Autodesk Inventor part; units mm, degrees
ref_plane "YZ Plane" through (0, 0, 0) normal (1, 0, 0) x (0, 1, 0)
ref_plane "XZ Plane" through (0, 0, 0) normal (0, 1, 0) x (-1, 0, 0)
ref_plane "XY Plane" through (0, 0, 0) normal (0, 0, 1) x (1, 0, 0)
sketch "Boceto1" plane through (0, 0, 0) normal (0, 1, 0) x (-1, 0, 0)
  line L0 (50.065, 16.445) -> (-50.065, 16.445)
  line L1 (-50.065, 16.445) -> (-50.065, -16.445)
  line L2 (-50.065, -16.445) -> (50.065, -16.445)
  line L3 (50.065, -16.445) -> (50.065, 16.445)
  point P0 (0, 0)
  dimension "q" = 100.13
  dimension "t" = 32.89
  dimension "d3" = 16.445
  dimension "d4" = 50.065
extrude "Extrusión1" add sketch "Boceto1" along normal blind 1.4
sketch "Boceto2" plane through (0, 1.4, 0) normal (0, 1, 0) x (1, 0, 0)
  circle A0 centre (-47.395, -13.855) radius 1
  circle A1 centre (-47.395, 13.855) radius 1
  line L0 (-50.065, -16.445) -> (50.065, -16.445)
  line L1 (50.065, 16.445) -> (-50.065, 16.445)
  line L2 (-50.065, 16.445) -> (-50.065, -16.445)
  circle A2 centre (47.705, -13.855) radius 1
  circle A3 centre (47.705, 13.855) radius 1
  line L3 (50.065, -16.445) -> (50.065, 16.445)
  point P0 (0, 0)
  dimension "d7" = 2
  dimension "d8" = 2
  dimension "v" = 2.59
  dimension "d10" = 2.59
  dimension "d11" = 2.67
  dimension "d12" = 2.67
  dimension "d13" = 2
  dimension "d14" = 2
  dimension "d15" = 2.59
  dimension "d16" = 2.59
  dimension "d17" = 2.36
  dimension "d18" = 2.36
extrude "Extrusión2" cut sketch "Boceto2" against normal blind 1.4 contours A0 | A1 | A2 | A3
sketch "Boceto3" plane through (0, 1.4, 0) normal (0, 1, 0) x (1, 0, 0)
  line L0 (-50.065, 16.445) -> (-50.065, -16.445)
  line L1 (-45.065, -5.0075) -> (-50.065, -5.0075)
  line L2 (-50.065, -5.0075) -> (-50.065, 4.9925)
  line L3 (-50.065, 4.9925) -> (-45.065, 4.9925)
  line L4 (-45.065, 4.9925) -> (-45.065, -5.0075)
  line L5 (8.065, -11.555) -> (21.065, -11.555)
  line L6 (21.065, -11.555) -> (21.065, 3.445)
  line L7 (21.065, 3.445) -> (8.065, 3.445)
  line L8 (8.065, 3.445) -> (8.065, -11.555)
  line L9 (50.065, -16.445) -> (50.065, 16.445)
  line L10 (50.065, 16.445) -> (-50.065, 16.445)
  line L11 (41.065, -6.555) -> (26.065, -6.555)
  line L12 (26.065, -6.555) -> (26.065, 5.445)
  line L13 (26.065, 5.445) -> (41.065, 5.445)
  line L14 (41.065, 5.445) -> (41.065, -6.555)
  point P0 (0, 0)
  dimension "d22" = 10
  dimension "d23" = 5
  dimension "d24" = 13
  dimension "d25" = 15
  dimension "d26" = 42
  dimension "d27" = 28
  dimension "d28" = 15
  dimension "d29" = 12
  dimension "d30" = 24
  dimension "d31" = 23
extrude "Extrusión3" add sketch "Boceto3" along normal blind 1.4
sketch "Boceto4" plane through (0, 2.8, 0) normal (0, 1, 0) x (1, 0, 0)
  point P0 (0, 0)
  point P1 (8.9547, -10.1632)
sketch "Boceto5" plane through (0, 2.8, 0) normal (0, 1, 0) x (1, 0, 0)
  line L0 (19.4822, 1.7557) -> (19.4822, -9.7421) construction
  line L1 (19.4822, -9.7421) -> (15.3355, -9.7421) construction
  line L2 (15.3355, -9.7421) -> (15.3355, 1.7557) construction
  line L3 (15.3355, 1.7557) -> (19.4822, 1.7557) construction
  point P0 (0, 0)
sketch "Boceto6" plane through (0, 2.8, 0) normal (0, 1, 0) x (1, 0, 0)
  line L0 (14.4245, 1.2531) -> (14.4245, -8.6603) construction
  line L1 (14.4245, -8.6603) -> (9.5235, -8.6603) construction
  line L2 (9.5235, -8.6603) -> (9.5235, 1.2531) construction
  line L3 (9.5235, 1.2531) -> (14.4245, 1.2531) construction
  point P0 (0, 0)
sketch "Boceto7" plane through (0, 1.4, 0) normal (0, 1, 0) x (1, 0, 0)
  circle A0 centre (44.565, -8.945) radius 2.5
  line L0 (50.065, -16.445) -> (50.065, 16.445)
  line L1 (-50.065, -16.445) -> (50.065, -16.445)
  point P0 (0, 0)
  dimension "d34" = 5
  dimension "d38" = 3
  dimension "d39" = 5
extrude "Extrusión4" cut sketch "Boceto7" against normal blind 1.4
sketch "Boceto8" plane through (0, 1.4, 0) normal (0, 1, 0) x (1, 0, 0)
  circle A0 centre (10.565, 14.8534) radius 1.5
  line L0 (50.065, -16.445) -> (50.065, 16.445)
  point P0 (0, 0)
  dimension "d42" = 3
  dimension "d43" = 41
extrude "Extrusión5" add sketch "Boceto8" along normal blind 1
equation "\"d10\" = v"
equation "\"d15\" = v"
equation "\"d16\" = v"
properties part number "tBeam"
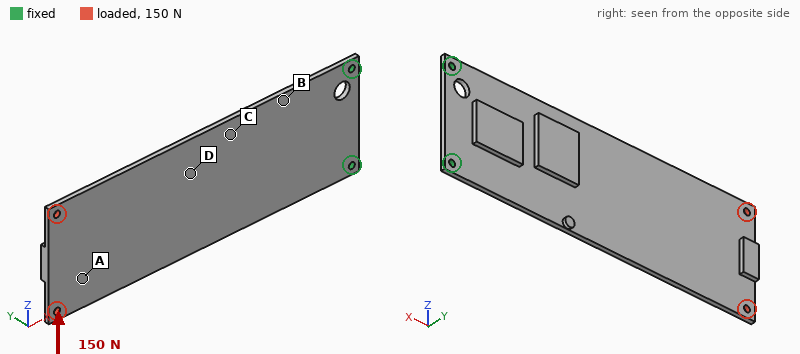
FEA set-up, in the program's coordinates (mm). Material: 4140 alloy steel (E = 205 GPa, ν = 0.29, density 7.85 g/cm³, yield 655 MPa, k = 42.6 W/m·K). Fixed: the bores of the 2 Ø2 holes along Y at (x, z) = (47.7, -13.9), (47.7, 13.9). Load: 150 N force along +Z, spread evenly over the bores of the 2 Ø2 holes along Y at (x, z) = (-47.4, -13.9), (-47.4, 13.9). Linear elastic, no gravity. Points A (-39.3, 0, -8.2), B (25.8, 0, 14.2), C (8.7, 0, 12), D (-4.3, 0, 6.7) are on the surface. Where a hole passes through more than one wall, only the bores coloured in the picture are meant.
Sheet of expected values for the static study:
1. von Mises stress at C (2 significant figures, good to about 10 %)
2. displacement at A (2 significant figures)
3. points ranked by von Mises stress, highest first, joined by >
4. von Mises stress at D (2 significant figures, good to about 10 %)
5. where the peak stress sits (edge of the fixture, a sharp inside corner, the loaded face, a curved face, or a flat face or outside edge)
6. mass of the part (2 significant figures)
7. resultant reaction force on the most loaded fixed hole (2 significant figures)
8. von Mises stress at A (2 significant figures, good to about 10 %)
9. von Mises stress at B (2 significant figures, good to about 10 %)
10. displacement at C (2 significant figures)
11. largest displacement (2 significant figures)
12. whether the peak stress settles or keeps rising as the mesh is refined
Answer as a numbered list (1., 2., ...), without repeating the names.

1. 27 MPa
2. 54 µm
3. B > C > D > A
4. 13 MPa
5. edge of the fixture
6. 41 g
7. 520 N
8. 7.2 MPa
9. 37 MPa
10. 16 µm
11. 66 µm
12. keeps rising
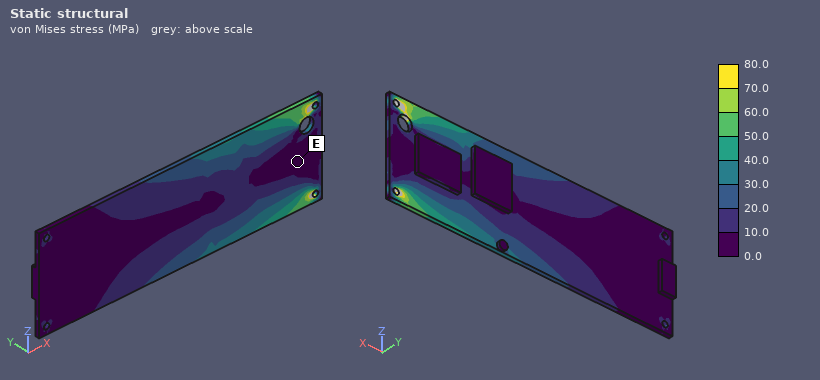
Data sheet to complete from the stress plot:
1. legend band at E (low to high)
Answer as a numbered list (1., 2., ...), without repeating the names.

1. 0.0 to 10.0 MPa
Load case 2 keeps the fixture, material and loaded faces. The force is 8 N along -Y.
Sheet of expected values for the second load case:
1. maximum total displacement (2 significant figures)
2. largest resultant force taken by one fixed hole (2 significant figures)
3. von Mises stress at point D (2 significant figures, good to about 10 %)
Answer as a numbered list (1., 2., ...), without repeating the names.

1. 1.3 mm
2. 8.8 N
3. 30 MPa
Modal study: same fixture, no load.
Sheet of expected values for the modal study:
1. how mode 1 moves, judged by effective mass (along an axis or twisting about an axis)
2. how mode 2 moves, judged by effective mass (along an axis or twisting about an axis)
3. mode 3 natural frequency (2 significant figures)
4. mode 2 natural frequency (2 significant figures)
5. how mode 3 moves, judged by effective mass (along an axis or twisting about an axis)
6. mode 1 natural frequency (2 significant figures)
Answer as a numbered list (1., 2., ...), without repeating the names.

1. along Y
2. along Y
3. 940 Hz
4. 710 Hz
5. twisting about X
6. 130 Hz
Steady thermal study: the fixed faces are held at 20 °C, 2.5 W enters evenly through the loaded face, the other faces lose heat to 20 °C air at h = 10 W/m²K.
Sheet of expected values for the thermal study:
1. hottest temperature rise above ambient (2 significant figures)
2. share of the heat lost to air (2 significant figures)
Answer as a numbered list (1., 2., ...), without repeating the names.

1. 71 K
2. 71 %
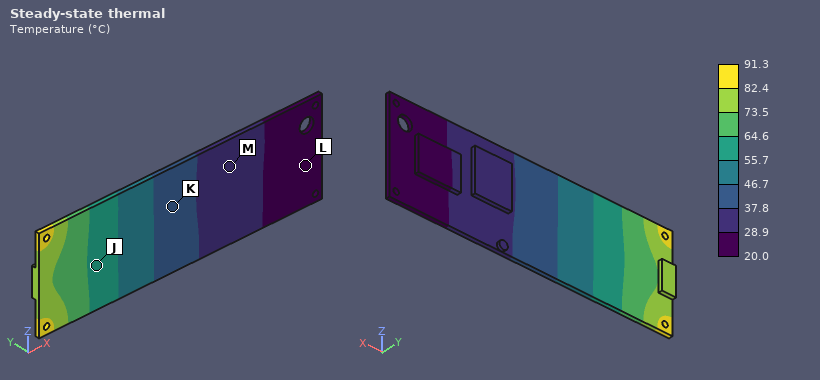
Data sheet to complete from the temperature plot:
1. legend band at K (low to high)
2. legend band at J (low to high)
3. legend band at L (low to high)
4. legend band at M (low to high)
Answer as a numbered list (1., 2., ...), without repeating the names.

1. 37.8 to 46.7 °C
2. 55.7 to 64.6 °C
3. 20.0 to 28.9 °C
4. 28.9 to 37.8 °C
